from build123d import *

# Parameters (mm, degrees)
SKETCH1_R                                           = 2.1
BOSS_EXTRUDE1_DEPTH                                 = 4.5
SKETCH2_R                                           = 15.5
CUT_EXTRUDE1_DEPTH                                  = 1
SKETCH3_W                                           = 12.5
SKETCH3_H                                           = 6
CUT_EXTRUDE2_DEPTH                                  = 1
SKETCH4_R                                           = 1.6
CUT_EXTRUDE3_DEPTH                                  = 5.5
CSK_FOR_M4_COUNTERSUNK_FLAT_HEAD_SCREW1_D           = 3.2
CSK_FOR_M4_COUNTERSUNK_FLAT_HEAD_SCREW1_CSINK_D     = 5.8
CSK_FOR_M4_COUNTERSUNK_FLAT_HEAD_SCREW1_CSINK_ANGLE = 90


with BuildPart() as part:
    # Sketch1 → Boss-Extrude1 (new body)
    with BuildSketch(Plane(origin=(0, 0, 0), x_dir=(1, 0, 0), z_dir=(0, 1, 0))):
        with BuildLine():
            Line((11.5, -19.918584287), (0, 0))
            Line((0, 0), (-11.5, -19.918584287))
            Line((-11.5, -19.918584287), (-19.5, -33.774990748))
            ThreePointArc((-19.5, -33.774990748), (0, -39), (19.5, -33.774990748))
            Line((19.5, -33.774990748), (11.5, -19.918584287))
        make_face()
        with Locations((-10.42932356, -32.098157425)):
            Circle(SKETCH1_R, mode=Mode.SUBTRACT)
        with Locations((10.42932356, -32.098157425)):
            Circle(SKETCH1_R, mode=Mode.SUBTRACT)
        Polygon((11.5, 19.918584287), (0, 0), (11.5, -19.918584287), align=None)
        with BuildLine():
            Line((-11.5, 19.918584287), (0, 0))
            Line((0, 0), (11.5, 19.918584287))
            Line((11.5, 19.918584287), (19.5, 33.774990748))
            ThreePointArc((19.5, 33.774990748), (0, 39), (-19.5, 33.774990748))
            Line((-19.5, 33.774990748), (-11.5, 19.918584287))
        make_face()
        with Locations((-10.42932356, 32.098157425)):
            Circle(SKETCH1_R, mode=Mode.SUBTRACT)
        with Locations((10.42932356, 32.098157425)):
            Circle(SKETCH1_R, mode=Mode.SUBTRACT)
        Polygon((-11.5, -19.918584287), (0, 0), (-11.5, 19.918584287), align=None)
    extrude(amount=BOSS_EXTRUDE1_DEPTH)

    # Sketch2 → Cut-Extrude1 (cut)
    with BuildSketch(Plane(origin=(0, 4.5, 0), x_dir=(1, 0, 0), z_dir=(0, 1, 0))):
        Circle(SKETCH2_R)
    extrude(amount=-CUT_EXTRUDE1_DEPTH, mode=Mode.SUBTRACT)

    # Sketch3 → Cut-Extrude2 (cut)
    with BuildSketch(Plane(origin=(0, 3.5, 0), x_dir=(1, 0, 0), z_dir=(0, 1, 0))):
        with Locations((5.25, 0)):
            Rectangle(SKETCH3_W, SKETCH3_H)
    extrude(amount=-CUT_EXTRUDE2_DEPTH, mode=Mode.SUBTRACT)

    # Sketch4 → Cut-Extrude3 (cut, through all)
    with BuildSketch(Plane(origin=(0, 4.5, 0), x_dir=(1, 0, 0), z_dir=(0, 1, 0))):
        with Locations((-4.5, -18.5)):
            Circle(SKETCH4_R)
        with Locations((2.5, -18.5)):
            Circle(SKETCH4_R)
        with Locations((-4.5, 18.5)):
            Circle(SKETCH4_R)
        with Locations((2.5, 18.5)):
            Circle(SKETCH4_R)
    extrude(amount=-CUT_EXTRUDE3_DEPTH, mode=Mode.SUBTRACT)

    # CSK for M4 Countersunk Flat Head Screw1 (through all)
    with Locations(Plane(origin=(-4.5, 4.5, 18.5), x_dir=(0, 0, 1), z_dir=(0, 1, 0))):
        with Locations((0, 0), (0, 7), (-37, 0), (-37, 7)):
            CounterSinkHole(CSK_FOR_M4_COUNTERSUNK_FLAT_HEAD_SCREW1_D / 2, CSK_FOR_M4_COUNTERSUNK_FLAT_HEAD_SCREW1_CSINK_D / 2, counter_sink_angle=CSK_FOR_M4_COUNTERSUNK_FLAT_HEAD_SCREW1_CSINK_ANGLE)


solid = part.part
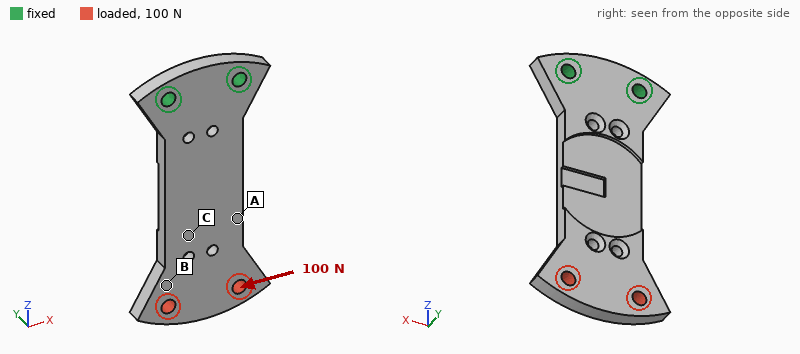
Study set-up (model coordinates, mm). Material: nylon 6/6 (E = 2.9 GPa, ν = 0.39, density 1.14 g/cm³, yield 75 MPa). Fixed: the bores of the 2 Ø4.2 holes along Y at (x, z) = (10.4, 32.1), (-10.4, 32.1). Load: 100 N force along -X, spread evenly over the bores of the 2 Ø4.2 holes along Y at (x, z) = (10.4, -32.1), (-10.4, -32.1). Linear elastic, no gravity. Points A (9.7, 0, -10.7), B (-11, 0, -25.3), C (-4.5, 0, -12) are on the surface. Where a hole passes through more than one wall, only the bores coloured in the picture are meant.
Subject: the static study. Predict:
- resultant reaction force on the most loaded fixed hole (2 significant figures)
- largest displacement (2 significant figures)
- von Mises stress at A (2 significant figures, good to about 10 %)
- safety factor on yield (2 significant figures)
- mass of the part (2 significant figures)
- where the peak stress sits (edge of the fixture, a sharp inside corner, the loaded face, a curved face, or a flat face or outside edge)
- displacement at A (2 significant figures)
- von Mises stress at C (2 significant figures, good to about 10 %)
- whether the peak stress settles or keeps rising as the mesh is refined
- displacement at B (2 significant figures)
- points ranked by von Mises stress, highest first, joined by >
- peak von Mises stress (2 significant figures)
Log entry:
290 N
0.93 mm
5.6 MPa
3.6
9.2 g
a flat face or outside edge
0.36 mm
3.9 MPa
settles
0.67 mm
A > C > B
21 MPa
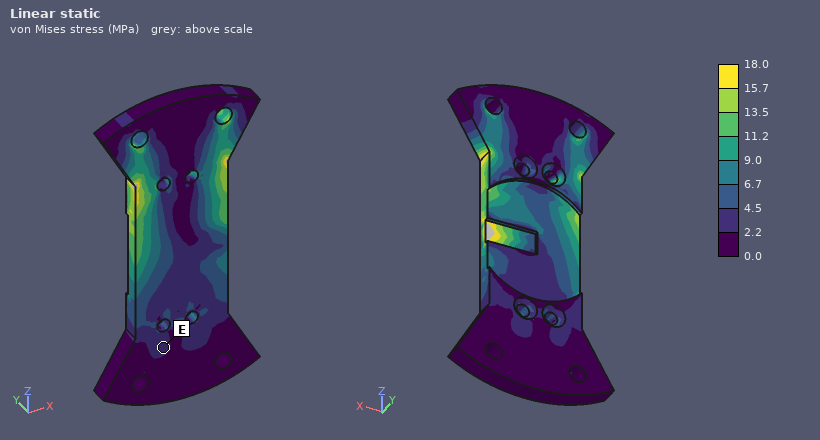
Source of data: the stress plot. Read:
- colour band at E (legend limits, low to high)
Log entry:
2.2 to 4.5 MPa
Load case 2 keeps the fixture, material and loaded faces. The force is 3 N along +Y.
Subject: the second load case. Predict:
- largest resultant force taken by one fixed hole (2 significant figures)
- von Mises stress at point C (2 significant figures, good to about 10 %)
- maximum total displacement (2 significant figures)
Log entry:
1.6 N
1.2 MPa
0.92 mm
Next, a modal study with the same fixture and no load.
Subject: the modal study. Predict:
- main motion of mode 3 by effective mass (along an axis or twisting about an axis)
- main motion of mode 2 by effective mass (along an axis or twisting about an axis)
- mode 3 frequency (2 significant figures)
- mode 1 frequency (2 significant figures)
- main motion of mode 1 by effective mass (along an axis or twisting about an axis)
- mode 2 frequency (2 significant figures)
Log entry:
along X
twisting about Z
1100 Hz
180 Hz
along Y
800 Hz
